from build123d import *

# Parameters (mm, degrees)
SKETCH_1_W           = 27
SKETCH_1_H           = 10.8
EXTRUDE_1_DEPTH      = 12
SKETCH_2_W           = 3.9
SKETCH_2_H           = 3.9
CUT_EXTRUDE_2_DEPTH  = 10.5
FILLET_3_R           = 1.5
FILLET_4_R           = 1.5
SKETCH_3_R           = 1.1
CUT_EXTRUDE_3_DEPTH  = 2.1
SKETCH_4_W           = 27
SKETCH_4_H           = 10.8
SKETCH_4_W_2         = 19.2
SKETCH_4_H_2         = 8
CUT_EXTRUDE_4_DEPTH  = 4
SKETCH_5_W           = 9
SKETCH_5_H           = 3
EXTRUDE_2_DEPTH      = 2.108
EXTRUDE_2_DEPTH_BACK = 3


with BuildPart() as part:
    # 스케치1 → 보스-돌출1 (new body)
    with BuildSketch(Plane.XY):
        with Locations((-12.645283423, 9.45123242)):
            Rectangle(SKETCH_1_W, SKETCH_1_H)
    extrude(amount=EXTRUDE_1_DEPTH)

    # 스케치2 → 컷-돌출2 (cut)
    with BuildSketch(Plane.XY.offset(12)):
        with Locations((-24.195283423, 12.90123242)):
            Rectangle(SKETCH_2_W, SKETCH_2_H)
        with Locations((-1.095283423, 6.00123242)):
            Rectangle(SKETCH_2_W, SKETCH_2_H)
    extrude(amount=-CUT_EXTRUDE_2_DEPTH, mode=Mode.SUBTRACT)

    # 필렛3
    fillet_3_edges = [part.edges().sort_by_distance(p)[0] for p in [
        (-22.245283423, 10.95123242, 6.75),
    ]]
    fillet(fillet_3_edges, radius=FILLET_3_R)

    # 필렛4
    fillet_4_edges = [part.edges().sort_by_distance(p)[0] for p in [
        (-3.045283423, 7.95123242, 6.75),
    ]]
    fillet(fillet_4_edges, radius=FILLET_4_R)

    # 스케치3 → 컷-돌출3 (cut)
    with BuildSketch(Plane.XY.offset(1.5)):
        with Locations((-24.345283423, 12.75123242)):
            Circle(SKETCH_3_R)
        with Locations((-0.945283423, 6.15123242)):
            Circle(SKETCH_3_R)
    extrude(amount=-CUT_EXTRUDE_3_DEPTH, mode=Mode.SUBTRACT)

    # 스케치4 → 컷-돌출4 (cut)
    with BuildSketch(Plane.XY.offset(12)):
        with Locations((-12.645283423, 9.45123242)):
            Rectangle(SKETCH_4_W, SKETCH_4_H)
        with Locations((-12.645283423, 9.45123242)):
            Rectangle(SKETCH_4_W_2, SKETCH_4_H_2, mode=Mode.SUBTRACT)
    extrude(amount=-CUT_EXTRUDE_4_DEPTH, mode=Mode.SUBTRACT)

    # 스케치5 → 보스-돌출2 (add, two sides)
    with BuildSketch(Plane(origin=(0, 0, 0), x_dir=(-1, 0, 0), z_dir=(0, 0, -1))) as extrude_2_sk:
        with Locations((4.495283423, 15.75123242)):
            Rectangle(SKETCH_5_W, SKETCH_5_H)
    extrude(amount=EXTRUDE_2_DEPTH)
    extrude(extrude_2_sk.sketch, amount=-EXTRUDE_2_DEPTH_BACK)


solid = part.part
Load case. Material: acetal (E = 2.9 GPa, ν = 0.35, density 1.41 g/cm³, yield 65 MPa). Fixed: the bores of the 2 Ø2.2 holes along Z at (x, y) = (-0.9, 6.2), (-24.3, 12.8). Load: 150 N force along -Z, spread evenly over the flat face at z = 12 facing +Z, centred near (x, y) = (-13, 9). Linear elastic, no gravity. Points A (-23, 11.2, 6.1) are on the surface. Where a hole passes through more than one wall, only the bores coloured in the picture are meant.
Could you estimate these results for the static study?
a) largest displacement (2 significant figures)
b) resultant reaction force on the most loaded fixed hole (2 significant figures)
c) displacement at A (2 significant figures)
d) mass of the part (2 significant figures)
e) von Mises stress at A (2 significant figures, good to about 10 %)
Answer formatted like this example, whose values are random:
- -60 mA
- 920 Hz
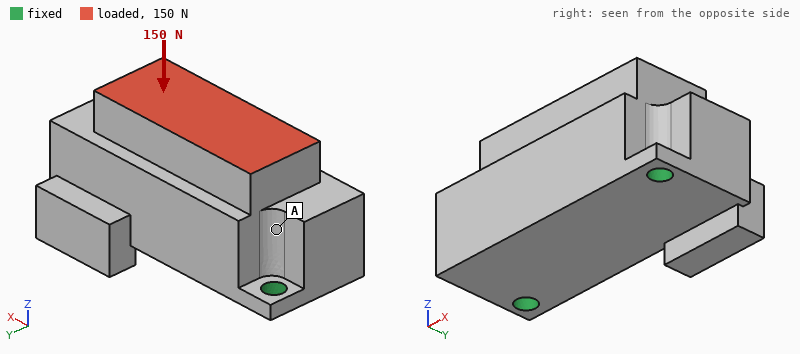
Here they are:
- 35 µm
- 83 N
- 25 µm
- 4.0 g
- 4.2 MPa
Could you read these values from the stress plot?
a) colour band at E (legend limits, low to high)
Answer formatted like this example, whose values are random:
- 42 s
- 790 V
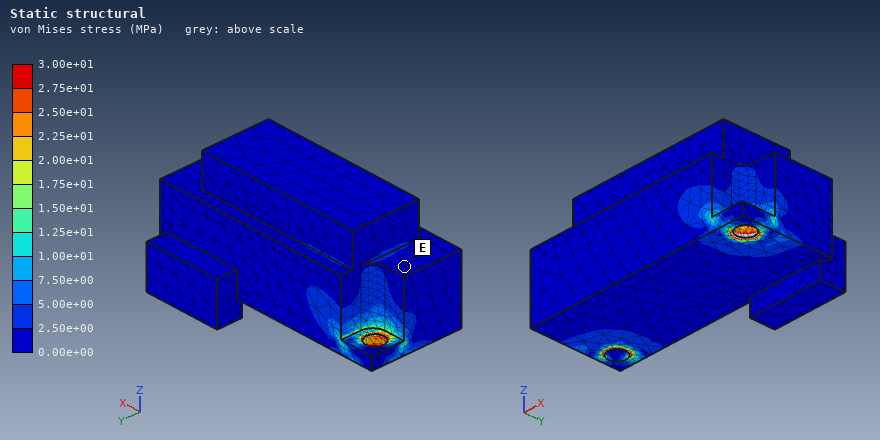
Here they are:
- 0.00e+00 to 2.50e+00 MPa
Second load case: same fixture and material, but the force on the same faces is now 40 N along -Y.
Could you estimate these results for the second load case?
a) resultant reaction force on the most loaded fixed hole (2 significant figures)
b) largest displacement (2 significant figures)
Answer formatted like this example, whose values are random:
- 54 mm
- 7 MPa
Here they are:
- 22 N
- 0.40 mm
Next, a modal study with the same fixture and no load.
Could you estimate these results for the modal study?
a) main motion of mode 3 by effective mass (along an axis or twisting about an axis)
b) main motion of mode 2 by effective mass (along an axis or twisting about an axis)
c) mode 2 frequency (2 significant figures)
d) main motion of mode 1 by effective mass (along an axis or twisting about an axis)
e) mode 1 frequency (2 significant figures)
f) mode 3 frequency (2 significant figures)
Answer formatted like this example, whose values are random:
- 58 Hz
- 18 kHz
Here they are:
- along X
- along Z
- 5600 Hz
- along Y
- 1400 Hz
- 7300 Hz
